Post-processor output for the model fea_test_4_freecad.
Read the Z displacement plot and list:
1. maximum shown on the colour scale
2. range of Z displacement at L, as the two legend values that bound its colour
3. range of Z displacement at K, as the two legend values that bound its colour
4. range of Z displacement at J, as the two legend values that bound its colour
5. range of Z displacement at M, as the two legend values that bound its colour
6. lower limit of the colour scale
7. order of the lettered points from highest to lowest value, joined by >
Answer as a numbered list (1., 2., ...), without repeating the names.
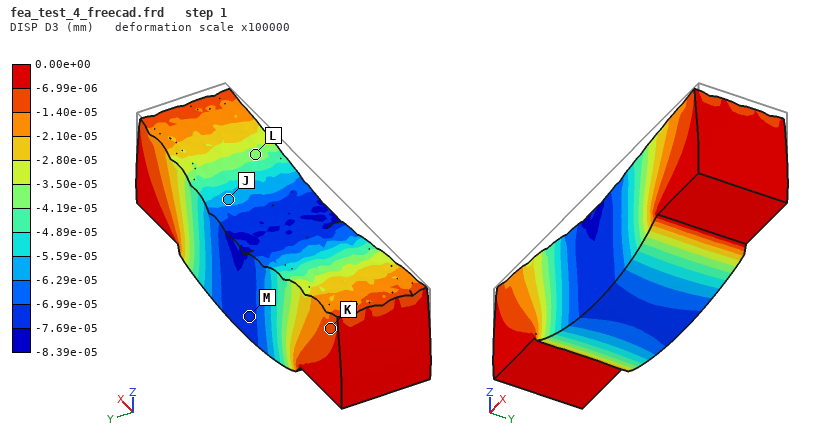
1. 0.00e+00 mm
2. -4.19e-05 to -3.50e-05 mm
3. -1.40e-05 to -6.99e-06 mm
4. -6.29e-05 to -5.59e-05 mm
5. -7.69e-05 to -6.99e-05 mm
6. -8.39e-05 mm
7. K > L > J > M
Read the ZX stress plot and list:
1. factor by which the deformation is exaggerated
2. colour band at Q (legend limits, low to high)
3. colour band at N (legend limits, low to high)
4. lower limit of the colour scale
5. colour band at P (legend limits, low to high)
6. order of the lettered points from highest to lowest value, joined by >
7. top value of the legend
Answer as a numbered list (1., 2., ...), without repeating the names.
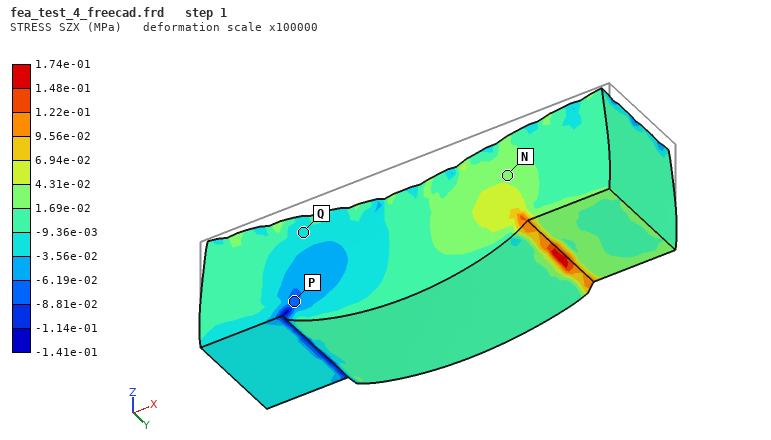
1. 100000
2. -3.56e-02 to -9.36e-03 MPa
3. 1.69e-02 to 4.31e-02 MPa
4. -1.41e-01 MPa
5. -8.81e-02 to -6.19e-02 MPa
6. N > Q > P
7. 1.74e-01 MPa
